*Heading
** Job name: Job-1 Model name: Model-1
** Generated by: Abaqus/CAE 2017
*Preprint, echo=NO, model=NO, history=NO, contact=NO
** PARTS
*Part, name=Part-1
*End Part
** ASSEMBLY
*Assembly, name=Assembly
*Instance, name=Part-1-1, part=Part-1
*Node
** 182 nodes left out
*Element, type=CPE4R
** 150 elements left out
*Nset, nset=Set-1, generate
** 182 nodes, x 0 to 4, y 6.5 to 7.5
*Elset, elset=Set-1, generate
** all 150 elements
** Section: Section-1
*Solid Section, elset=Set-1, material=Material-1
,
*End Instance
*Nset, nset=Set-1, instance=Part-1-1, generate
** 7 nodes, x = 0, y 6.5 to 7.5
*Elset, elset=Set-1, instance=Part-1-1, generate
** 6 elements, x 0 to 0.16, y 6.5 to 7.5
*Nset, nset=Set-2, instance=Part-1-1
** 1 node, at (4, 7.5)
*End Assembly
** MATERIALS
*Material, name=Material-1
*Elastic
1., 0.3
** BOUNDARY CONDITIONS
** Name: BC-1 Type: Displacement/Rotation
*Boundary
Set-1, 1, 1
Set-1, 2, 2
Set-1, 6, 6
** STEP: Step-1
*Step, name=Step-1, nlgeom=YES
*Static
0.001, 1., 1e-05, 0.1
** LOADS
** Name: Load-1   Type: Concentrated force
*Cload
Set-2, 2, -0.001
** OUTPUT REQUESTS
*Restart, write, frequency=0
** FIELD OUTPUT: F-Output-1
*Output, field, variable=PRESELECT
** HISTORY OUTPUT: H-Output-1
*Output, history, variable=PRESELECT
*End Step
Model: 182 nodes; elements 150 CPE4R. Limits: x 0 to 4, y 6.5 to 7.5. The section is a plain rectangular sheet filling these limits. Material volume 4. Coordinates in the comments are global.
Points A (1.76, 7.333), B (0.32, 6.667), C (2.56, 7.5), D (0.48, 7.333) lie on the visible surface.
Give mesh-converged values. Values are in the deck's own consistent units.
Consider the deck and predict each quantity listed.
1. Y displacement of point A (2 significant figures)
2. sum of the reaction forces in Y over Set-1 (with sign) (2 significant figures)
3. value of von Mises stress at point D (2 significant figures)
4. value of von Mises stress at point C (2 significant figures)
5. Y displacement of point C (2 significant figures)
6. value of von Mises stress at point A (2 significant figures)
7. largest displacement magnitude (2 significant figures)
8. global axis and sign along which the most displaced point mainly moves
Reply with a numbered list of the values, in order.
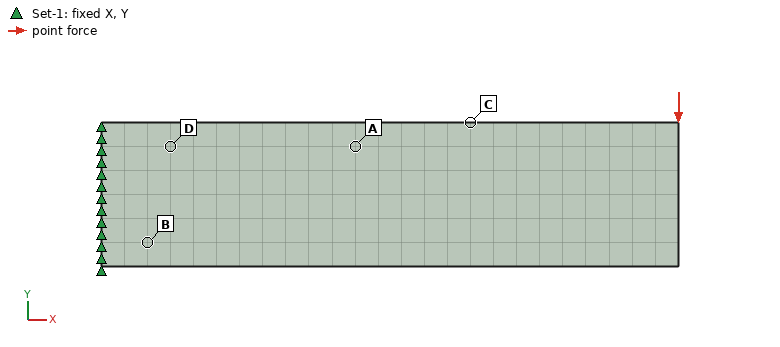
1. -0.064
2. 0.0010
3. 0.013
4. 0.0081
5. -0.12
6. 0.0084
7. 0.26
8. -Y
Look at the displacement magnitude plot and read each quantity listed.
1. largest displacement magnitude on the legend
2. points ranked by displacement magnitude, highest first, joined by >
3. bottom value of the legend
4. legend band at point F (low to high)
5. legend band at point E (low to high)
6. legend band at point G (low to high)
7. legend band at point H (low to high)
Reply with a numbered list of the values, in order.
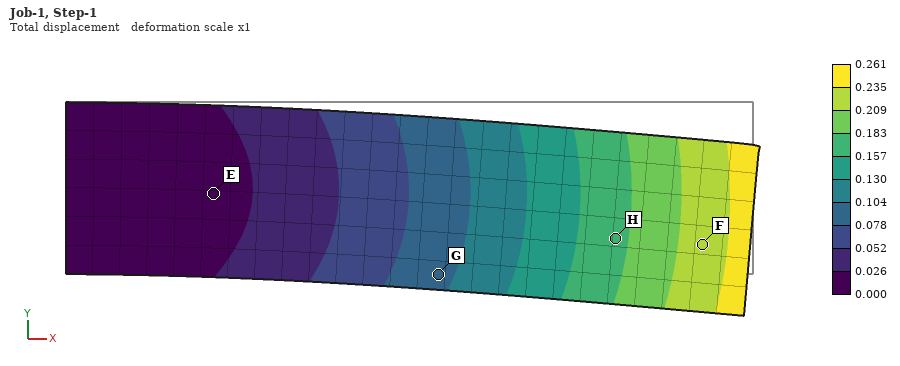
1. 0.261
2. F > H > G > E
3. 0.000
4. 0.209 to 0.235
5. 0.000 to 0.026
6. 0.078 to 0.104
7. 0.157 to 0.183
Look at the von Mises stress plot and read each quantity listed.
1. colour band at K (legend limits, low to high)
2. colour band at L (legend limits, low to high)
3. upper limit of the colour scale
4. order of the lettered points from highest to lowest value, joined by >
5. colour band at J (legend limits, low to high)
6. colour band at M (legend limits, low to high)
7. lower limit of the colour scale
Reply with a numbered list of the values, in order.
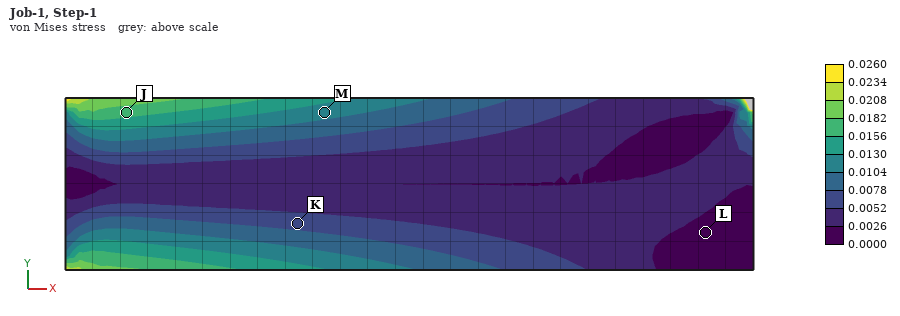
1. 0.0052 to 0.0078
2. 0.0000 to 0.0026
3. 0.0260
4. J > M > K > L
5. 0.0156 to 0.0182
6. 0.0104 to 0.0130
7. 0.0000
